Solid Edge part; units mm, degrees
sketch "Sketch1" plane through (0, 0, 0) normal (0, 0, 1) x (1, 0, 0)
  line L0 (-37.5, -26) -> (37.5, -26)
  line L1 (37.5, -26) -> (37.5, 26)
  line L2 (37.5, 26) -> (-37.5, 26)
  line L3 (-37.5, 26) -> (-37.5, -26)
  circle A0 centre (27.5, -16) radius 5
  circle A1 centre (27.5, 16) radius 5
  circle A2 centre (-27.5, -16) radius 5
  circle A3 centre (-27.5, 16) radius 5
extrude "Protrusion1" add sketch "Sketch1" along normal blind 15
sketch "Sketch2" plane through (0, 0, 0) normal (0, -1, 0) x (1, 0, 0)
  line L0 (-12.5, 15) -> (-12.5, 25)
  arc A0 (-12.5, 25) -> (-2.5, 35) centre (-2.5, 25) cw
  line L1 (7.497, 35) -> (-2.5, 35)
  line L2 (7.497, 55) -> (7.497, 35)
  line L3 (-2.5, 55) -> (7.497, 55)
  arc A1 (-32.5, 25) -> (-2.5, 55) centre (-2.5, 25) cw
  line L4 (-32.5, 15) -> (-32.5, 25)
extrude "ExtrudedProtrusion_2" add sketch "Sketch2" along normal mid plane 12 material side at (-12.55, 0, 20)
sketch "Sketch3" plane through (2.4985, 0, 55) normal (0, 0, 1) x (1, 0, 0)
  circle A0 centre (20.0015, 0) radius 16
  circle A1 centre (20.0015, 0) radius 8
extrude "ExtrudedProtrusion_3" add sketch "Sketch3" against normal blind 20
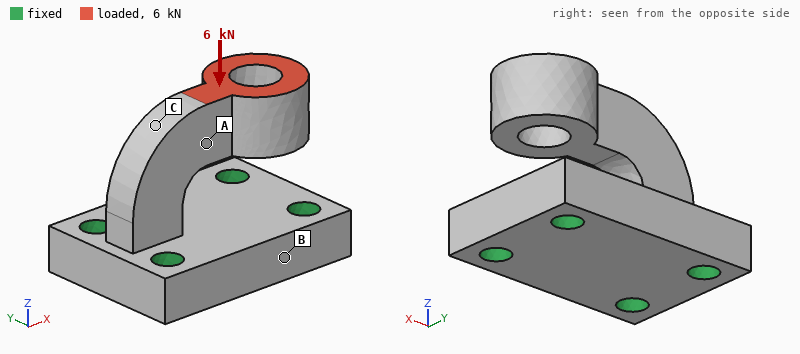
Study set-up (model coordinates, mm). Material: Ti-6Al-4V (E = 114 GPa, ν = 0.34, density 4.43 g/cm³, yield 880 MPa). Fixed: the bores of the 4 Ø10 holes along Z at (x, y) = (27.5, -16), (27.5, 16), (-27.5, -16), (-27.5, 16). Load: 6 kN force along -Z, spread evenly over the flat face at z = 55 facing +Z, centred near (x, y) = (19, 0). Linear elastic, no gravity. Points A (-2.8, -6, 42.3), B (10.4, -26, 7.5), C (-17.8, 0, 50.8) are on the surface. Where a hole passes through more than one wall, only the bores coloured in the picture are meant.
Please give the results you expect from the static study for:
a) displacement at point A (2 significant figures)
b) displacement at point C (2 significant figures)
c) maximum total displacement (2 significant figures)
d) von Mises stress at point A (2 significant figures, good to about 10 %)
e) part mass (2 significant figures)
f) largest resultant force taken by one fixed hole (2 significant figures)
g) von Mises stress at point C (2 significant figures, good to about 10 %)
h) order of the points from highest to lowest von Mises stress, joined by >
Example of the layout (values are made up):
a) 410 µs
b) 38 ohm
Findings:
a) 0.25 mm
b) 0.25 mm
c) 0.82 mm
d) 84 MPa
e) 350 g
f) 1.7 kN
g) 170 MPa
h) C > A > B
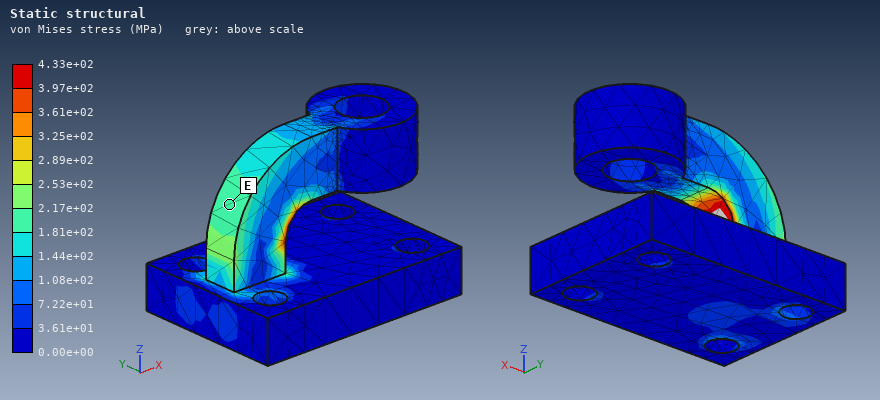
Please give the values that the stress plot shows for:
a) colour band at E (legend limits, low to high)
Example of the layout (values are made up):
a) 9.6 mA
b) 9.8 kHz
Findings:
a) 1.81e+02 to 2.17e+02 MPa
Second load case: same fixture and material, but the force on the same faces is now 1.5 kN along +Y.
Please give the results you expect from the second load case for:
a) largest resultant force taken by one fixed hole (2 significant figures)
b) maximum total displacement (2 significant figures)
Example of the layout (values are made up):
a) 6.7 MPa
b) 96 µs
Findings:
a) 2.9 kN
b) 0.57 mm
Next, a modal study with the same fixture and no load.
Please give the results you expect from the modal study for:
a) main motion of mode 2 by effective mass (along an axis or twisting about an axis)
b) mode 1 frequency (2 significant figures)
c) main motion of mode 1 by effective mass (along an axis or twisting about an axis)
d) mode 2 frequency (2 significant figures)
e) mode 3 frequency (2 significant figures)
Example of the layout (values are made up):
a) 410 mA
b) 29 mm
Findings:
a) along Z
b) 1200 Hz
c) along Y
d) 1900 Hz
e) 3900 Hz
